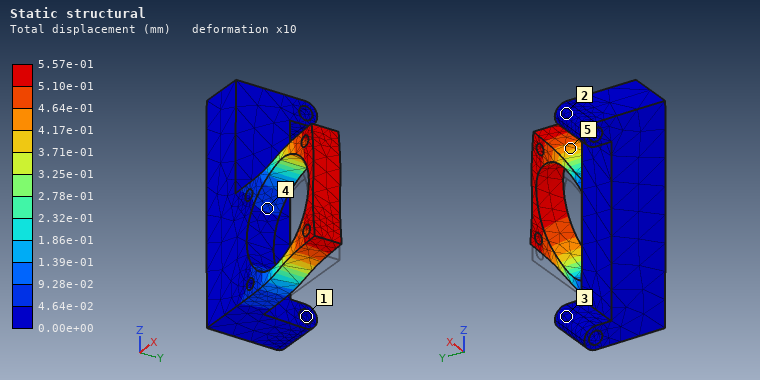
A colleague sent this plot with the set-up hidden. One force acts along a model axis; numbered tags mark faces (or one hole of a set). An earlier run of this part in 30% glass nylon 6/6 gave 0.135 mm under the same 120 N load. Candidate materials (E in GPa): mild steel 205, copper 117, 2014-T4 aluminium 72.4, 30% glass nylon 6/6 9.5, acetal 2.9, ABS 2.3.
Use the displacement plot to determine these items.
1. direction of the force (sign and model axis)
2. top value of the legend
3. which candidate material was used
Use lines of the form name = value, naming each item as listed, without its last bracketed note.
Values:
direction of the force = +Z
top value of the legend = 5.57e-01 mm
which candidate material was used = ABS
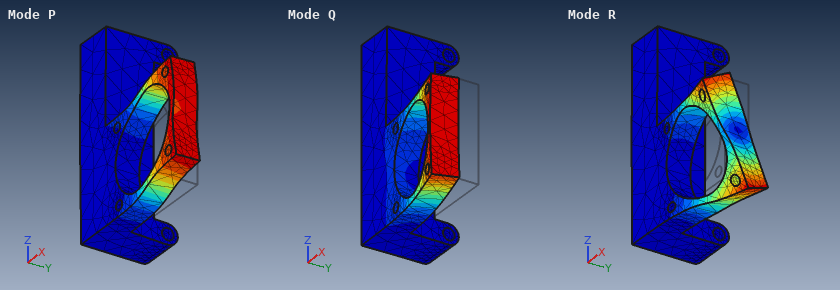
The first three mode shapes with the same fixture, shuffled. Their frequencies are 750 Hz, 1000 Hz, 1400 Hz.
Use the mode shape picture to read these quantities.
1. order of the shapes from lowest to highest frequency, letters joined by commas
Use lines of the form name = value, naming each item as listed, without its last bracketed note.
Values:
order of the shapes from lowest to highest frequency, letters joined by commas = Q, P, R
